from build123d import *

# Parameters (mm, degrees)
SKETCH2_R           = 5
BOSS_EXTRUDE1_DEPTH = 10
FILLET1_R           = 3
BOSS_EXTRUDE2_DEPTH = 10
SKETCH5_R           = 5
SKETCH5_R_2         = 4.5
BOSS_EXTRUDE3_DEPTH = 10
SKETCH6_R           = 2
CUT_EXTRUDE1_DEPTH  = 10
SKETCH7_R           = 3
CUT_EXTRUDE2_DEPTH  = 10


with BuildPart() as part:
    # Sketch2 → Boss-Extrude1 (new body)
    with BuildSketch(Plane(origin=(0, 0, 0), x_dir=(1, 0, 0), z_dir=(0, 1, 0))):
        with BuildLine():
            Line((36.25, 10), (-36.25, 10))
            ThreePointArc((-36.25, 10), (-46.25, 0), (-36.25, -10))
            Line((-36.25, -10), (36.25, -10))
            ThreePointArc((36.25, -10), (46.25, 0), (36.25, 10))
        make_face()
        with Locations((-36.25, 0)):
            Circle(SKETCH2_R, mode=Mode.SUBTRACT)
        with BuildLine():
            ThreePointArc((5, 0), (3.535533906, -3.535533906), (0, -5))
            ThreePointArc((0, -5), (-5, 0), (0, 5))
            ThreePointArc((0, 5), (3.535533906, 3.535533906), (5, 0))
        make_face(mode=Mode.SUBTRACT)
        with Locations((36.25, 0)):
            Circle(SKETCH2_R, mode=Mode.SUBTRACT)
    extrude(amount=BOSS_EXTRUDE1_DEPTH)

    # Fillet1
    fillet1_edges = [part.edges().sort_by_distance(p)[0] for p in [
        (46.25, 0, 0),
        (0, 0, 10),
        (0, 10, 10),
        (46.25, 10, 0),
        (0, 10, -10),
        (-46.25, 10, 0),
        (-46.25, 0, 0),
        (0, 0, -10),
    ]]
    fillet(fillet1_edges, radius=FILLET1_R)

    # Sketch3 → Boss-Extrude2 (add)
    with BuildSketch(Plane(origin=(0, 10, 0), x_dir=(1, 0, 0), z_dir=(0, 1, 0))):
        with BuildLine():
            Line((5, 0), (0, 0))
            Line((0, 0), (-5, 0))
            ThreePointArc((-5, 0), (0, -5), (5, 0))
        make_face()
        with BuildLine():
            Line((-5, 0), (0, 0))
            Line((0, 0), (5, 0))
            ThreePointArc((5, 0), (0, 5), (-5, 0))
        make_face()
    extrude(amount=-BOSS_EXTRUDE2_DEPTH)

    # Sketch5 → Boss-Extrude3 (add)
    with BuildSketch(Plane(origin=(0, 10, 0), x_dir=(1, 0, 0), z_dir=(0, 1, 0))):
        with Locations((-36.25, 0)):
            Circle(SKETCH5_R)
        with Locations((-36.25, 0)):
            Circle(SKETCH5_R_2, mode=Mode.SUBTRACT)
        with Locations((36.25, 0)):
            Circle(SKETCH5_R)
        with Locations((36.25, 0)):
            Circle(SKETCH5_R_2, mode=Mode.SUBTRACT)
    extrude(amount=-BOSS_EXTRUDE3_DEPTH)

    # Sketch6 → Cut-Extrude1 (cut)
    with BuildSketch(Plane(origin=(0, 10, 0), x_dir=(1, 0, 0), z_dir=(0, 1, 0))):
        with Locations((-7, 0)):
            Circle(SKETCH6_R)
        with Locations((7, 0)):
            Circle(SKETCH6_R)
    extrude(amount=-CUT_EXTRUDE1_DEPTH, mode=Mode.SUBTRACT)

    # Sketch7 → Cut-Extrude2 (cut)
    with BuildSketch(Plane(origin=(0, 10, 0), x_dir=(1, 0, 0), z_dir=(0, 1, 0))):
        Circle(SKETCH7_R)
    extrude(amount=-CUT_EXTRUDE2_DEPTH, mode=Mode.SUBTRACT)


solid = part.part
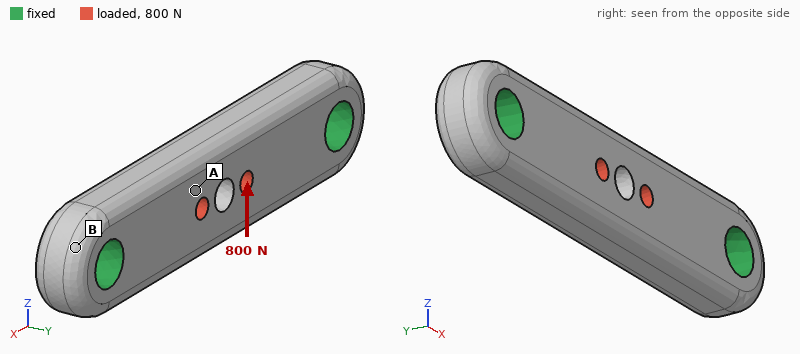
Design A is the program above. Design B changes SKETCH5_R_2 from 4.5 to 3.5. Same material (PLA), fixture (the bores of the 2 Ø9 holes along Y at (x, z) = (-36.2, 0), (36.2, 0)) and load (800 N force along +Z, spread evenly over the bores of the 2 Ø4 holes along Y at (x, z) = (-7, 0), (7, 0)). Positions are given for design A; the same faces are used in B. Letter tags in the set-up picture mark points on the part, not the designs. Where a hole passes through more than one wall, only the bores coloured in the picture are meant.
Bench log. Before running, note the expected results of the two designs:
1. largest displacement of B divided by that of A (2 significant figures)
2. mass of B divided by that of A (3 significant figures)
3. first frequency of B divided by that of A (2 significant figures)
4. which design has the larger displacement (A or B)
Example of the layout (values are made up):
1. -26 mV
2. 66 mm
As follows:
1. 1.2
2. 1.03
3. 0.93
4. B
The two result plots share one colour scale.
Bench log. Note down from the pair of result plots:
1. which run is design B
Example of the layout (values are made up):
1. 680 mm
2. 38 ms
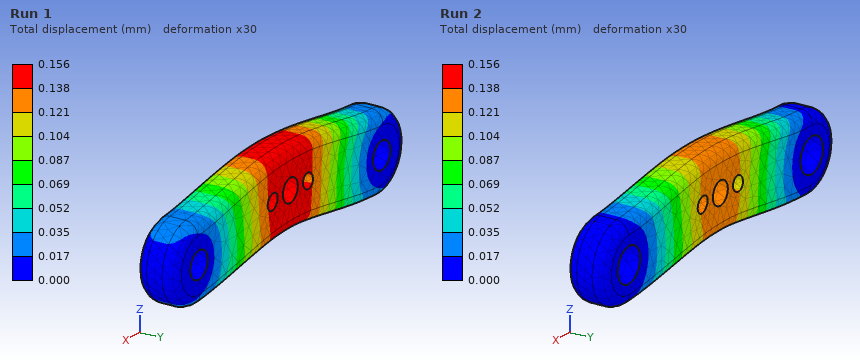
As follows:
1. Run 1
